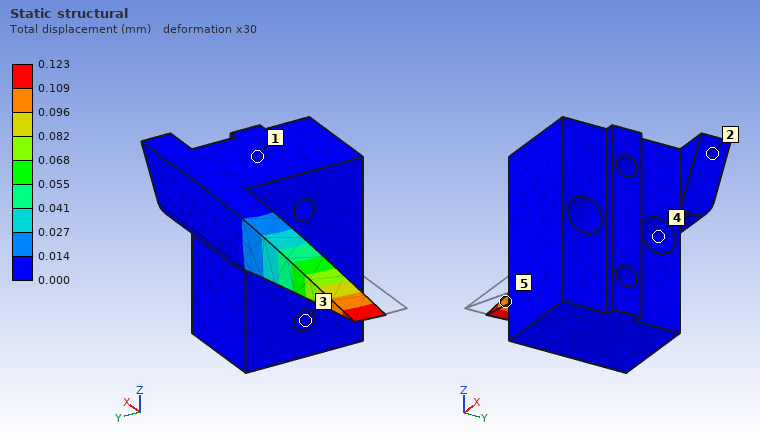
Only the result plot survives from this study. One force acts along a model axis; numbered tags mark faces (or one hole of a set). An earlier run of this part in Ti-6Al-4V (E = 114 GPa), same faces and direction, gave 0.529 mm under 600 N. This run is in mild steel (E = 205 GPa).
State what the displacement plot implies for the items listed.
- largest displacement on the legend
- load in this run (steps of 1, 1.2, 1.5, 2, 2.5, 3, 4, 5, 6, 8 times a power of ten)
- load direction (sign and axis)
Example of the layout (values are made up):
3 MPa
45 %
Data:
0.123 mm
250 N
+Y
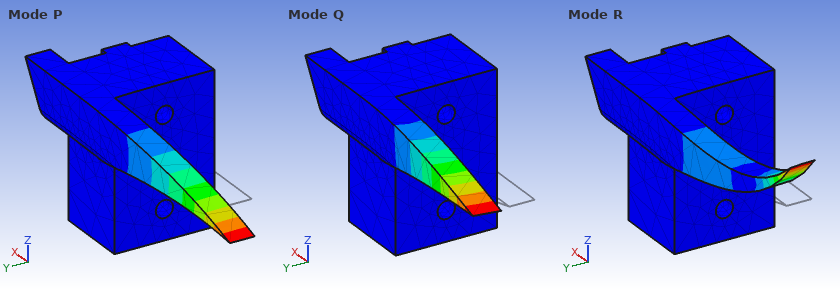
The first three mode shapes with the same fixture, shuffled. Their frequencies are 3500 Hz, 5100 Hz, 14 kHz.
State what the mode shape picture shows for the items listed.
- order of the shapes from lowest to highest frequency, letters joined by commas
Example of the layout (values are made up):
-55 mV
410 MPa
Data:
Q, P, R
